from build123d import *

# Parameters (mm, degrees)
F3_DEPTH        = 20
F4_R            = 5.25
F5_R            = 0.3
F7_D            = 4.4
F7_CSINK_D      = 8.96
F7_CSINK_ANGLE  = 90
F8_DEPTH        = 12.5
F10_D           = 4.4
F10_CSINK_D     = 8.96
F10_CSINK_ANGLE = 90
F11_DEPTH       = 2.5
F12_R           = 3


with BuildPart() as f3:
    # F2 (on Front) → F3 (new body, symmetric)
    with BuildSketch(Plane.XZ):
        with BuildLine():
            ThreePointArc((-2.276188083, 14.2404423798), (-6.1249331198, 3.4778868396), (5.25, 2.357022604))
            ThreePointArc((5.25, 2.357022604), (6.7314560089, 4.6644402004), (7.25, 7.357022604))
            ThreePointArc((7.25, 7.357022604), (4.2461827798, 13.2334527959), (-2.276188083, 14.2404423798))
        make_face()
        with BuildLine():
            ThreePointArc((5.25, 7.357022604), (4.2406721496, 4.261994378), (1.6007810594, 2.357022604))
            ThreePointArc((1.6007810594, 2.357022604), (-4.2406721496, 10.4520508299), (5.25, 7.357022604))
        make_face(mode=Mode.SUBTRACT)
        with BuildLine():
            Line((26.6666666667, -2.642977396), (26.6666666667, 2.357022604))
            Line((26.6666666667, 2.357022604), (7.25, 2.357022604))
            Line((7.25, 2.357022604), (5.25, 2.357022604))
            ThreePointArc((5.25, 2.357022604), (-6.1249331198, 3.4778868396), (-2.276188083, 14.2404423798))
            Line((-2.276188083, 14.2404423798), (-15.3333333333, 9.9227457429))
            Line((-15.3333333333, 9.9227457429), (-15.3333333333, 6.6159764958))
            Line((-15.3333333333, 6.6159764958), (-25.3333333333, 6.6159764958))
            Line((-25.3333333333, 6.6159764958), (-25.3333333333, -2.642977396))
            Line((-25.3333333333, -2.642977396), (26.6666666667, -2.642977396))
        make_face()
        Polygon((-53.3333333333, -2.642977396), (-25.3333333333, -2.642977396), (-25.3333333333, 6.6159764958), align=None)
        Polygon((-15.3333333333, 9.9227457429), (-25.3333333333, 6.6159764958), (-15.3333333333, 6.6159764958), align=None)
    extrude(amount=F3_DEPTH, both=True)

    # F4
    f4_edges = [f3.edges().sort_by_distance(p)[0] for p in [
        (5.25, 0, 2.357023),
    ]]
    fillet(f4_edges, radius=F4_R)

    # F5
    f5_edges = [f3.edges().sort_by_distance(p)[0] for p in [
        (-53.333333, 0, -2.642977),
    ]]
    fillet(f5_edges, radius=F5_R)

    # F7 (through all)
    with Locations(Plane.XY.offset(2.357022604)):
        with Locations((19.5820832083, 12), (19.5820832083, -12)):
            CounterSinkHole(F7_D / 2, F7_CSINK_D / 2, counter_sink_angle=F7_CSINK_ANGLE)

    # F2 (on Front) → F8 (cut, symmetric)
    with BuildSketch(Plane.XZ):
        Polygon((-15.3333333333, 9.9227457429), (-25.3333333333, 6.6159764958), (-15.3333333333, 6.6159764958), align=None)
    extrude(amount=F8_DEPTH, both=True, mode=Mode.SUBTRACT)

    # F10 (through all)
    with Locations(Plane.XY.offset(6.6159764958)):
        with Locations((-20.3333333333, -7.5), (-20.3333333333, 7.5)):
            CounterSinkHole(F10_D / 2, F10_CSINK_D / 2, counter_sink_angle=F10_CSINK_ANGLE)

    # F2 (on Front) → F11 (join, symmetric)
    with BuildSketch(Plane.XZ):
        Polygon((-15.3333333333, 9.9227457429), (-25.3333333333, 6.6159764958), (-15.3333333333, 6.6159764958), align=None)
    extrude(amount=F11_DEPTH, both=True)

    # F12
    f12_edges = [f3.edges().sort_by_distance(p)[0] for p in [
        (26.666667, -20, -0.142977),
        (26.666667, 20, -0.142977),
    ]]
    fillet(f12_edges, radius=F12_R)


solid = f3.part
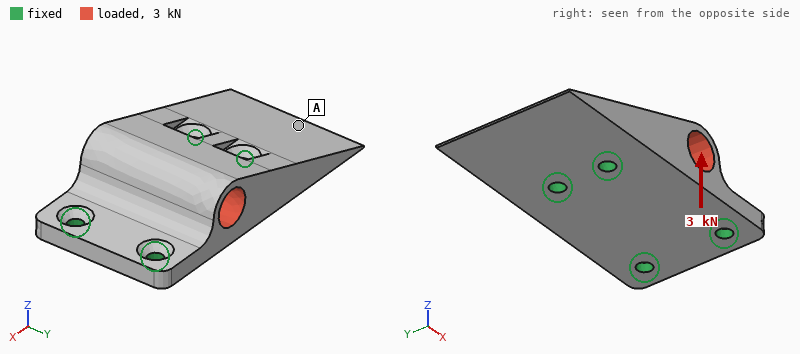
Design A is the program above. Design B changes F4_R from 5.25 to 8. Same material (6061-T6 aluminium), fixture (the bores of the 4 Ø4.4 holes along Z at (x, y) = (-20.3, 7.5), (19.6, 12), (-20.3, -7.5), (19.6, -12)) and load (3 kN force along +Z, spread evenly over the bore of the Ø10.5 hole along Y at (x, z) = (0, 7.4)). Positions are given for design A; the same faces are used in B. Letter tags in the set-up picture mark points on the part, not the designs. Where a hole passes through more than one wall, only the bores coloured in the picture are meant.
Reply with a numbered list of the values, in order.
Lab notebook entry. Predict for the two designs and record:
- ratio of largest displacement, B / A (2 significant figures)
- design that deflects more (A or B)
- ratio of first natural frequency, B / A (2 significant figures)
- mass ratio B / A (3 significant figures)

1. 0.90
2. A
3. 1.0
4. 1.01
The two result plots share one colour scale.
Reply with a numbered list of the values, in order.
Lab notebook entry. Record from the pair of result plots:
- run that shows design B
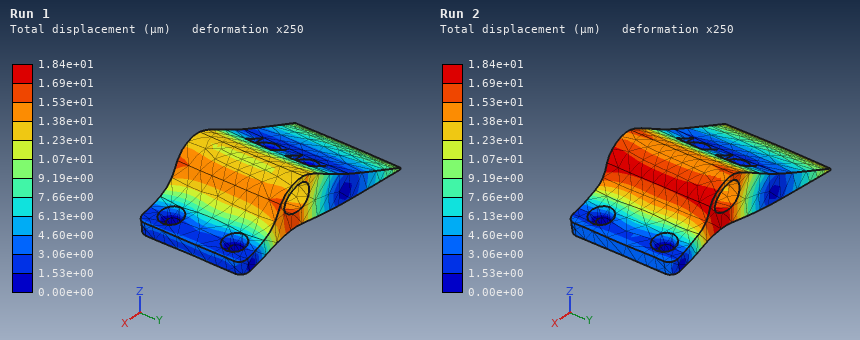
1. Run 1
